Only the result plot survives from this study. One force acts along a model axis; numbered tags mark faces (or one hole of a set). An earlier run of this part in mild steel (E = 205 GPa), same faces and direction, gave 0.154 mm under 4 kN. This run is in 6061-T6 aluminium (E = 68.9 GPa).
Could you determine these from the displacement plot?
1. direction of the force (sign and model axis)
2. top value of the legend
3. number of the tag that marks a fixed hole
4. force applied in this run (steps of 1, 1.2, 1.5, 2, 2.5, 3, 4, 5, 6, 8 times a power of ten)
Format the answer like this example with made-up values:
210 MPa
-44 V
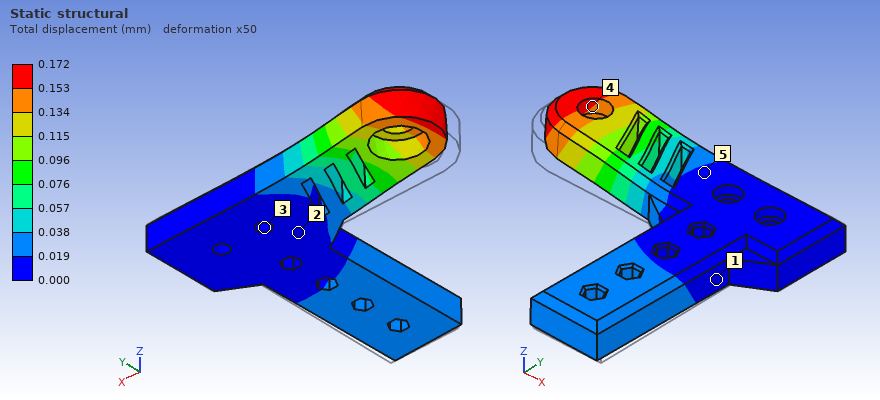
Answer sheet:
+Y
0.172 mm
3
1.5 kN
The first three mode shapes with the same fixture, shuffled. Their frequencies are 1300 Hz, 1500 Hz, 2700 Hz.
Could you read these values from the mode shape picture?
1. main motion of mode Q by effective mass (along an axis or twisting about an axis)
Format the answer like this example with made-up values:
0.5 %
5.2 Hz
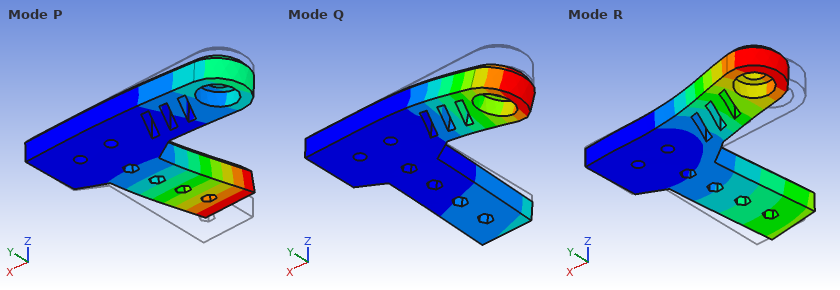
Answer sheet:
along Z
